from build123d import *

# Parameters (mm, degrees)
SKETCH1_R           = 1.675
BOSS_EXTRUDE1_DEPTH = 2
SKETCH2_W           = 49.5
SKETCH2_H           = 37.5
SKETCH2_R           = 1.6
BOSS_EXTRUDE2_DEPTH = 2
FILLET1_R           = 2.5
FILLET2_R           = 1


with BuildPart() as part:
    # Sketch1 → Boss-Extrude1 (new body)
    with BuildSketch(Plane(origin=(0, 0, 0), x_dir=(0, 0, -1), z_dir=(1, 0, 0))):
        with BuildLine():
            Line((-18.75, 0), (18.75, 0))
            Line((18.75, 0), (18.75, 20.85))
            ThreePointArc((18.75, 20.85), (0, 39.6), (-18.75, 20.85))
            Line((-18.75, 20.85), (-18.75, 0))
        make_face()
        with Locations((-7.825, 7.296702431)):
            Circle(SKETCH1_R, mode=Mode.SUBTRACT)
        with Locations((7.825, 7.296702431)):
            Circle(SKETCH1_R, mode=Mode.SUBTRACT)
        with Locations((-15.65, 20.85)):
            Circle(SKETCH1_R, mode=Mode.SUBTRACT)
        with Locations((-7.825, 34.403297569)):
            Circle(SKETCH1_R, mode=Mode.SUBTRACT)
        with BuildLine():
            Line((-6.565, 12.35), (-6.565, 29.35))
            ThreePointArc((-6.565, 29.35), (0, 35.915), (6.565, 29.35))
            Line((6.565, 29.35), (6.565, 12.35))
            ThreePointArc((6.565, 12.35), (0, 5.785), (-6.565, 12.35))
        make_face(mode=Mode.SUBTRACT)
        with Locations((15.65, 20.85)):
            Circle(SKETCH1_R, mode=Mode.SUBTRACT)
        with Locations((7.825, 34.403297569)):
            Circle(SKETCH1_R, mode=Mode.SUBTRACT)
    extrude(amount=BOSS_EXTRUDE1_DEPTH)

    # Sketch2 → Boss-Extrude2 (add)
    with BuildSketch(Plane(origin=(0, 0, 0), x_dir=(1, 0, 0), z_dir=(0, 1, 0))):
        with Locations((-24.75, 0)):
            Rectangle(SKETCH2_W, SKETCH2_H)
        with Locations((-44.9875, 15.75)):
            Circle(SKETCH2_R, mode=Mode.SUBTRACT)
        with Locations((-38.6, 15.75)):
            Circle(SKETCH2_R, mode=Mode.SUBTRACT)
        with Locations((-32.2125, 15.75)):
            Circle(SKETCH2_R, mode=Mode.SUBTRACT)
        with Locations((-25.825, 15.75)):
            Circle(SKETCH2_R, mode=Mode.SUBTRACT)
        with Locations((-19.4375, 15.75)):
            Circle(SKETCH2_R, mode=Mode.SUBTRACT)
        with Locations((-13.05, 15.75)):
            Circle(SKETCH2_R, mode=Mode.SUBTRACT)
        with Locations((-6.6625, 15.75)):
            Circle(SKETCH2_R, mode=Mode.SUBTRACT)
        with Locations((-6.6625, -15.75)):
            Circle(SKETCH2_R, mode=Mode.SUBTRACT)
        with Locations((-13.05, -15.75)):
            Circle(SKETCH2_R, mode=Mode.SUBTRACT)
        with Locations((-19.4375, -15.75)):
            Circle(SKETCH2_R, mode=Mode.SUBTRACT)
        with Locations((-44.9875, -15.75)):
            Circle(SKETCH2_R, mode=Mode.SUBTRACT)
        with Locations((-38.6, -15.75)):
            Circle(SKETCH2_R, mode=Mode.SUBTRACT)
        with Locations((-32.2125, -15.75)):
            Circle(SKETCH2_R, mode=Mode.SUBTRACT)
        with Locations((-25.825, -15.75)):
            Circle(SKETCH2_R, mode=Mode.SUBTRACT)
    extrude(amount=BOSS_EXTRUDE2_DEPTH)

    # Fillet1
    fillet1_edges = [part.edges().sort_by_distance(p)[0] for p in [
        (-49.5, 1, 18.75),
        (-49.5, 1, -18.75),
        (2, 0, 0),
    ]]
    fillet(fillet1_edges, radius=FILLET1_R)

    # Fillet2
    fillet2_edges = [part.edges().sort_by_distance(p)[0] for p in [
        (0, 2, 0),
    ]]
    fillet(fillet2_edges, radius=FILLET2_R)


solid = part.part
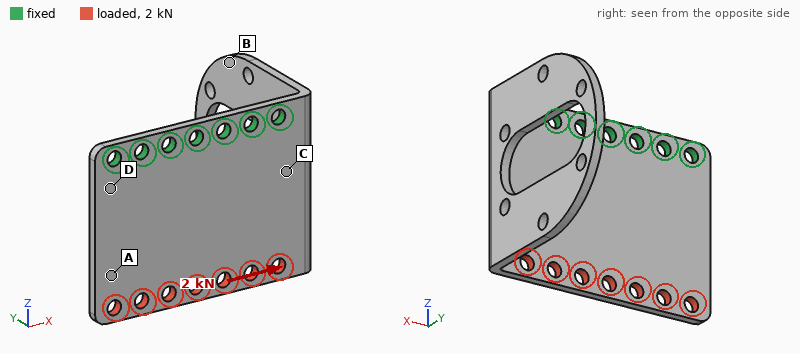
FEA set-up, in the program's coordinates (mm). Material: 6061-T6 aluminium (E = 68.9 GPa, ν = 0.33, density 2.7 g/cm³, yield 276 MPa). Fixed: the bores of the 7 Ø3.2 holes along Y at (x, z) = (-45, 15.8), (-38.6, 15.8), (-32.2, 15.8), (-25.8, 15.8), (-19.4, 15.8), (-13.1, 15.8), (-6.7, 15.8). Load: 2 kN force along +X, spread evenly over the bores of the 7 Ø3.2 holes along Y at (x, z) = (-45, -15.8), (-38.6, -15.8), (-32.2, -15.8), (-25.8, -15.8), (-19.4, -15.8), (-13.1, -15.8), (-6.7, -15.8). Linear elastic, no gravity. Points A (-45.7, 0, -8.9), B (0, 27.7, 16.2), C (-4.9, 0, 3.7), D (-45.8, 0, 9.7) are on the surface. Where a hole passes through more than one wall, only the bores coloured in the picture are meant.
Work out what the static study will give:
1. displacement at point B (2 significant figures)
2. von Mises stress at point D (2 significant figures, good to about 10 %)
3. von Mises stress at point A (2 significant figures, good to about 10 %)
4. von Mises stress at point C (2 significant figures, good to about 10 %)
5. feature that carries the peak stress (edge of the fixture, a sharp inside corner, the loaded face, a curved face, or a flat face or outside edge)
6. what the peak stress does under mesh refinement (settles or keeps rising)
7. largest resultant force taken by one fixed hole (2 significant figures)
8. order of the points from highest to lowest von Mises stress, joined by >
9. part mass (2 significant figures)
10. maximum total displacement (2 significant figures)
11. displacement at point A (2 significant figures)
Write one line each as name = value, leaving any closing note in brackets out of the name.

displacement at point B = 12 µm
von Mises stress at point D = 65 MPa
von Mises stress at point A = 22 MPa
von Mises stress at point C = 35 MPa
feature that carries the peak stress = edge of the fixture
what the peak stress does under mesh refinement = keeps rising
largest resultant force taken by one fixed hole = 1.3 kN
order of the points from highest to lowest von Mises stress, joined by > = D > C > A > B
part mass = 14 g
maximum total displacement = 58 µm
displacement at point A = 38 µm
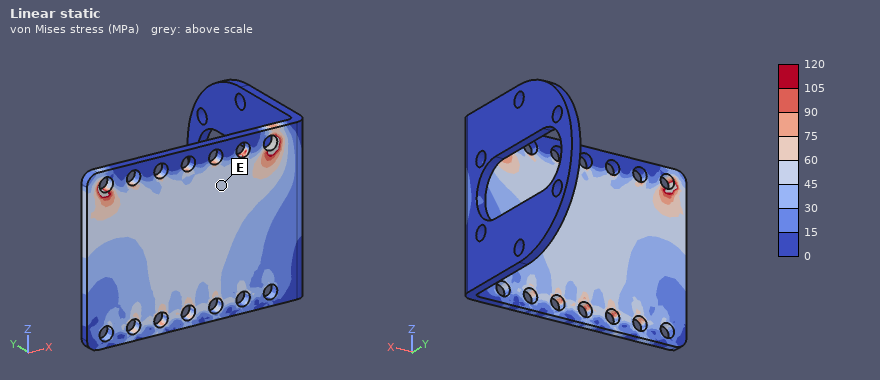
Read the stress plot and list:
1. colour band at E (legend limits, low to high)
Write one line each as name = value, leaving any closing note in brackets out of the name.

colour band at E = 45 to 60 MPa
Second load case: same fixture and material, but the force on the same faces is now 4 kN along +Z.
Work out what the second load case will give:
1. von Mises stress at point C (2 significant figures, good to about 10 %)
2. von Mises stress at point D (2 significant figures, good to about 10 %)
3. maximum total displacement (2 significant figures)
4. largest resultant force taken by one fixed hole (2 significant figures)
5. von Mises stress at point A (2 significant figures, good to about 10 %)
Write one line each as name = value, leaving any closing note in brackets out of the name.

von Mises stress at point C = 30 MPa
von Mises stress at point D = 45 MPa
maximum total displacement = 23 µm
largest resultant force taken by one fixed hole = 760 N
von Mises stress at point A = 37 MPa
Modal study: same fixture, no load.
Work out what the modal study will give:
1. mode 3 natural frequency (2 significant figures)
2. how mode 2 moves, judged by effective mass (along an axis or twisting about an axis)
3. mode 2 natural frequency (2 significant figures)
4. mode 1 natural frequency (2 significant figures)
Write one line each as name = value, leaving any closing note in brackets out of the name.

mode 3 natural frequency = 2100 Hz
how mode 2 moves, judged by effective mass = along Y
mode 2 natural frequency = 1200 Hz
mode 1 natural frequency = 920 Hz
